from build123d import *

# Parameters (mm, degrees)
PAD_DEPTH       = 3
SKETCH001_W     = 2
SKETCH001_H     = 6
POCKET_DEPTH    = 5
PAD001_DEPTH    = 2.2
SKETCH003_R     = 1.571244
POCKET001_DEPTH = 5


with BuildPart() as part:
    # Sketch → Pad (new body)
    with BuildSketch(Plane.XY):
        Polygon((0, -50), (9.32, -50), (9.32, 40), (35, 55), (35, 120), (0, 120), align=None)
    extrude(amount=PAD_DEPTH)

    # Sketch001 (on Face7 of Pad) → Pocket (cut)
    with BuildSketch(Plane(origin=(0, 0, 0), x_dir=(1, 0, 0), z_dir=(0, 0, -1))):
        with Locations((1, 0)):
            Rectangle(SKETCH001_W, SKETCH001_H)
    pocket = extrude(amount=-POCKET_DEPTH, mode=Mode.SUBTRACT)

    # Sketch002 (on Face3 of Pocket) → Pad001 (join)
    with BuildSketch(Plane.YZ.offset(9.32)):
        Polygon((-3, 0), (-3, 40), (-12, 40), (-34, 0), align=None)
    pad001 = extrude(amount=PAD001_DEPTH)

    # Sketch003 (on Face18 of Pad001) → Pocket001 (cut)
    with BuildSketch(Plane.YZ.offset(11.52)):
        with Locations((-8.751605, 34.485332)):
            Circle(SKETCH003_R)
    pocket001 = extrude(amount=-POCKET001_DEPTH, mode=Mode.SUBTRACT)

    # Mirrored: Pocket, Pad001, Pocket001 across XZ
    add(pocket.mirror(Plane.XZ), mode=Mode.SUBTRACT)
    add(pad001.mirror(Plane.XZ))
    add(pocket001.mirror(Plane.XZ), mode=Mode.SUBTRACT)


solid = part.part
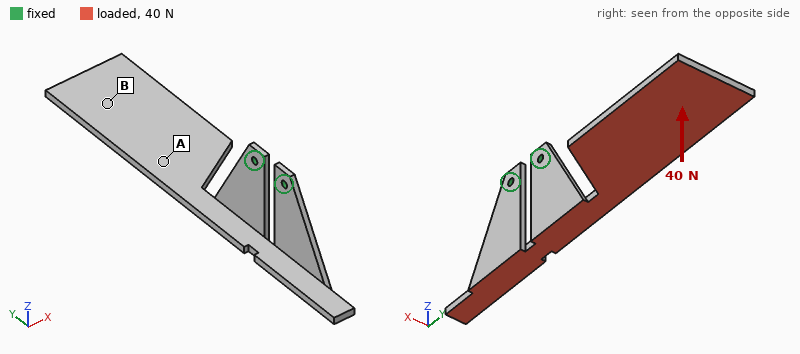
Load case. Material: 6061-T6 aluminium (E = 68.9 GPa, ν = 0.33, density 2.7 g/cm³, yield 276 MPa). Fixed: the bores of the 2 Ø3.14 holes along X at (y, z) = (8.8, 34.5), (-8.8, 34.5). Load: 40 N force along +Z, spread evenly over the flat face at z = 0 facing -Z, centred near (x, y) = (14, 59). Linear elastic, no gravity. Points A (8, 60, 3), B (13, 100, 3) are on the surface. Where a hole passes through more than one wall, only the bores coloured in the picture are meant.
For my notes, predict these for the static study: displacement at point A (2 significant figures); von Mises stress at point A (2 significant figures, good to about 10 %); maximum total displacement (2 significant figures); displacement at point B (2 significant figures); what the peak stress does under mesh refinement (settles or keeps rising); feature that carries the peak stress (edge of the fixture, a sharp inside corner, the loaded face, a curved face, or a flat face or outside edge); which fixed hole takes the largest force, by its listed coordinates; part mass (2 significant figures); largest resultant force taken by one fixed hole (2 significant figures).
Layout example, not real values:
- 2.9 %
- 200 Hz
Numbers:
- 0.48 mm
- 18 MPa
- 2.0 mm
- 1.4 mm
- keeps rising
- a sharp inside corner
- (8.8, 34.5)
- 37 g
- 81 N
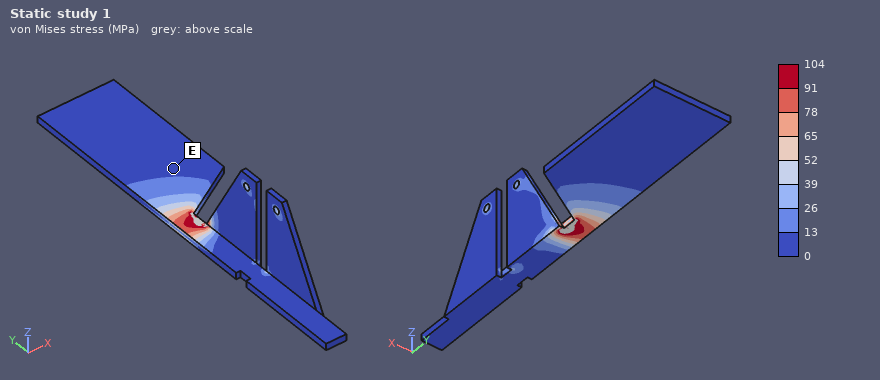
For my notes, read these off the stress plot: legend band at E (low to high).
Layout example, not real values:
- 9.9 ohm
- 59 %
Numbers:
- 0 to 13 MPa
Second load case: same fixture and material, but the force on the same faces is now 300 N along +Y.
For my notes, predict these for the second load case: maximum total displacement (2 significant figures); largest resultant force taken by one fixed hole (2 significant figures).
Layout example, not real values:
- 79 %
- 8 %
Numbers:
- 1.7 mm
- 220 N
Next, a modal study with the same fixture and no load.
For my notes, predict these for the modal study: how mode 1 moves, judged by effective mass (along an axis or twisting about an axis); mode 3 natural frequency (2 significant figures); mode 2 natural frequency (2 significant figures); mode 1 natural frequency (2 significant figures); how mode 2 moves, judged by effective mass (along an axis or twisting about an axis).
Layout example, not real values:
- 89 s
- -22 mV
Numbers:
- along X
- 490 Hz
- 160 Hz
- 140 Hz
- along Z
